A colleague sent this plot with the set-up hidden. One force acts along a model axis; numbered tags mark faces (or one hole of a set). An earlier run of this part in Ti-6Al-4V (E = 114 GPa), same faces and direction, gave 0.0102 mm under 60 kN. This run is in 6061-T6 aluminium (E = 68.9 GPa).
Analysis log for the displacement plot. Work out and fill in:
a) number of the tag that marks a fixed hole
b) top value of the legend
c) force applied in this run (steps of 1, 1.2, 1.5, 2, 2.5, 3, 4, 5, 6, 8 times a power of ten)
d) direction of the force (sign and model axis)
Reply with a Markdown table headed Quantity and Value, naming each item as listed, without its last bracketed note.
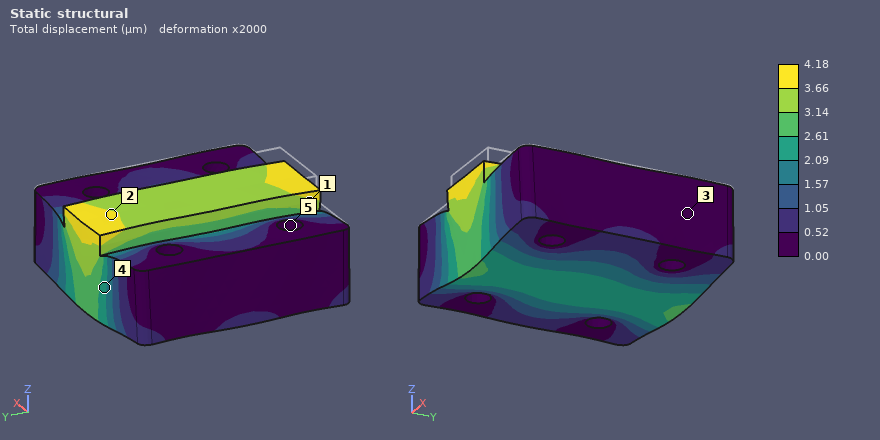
| Quantity | Value |
|---|---|
| number of the tag that marks a fixed hole | 5 |
| top value of the legend | 4.18 µm |
| force applied in this run | 15 kN |
| direction of the force | -Z |
